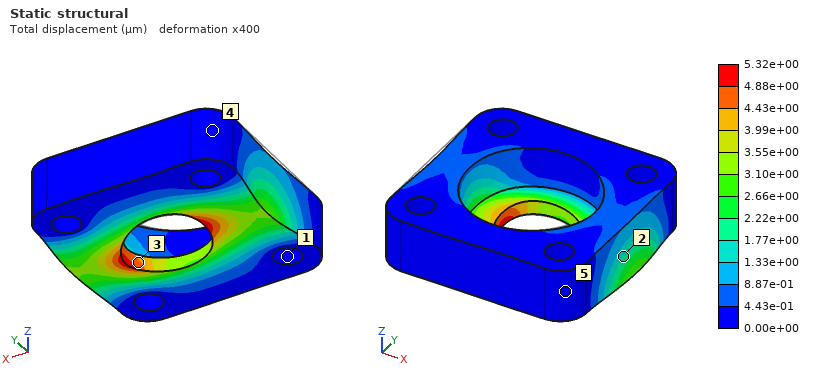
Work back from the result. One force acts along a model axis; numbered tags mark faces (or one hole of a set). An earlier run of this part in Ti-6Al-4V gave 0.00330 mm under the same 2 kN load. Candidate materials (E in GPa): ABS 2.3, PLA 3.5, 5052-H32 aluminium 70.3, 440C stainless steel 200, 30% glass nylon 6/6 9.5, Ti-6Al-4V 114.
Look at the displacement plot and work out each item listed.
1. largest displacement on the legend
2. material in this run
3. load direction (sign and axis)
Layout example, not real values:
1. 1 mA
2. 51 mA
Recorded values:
1. 5.32e+00 µm
2. 5052-H32 aluminium
3. +X
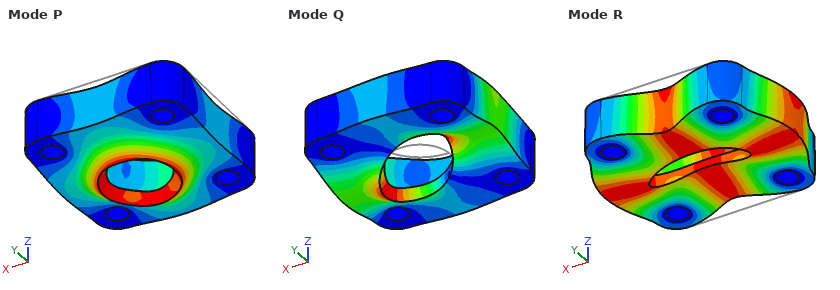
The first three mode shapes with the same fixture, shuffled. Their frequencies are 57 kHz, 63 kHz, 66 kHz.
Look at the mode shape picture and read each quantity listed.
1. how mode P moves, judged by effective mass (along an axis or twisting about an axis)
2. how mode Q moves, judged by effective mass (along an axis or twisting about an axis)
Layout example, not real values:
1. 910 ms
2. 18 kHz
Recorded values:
1. along Z
2. twisting about Y
